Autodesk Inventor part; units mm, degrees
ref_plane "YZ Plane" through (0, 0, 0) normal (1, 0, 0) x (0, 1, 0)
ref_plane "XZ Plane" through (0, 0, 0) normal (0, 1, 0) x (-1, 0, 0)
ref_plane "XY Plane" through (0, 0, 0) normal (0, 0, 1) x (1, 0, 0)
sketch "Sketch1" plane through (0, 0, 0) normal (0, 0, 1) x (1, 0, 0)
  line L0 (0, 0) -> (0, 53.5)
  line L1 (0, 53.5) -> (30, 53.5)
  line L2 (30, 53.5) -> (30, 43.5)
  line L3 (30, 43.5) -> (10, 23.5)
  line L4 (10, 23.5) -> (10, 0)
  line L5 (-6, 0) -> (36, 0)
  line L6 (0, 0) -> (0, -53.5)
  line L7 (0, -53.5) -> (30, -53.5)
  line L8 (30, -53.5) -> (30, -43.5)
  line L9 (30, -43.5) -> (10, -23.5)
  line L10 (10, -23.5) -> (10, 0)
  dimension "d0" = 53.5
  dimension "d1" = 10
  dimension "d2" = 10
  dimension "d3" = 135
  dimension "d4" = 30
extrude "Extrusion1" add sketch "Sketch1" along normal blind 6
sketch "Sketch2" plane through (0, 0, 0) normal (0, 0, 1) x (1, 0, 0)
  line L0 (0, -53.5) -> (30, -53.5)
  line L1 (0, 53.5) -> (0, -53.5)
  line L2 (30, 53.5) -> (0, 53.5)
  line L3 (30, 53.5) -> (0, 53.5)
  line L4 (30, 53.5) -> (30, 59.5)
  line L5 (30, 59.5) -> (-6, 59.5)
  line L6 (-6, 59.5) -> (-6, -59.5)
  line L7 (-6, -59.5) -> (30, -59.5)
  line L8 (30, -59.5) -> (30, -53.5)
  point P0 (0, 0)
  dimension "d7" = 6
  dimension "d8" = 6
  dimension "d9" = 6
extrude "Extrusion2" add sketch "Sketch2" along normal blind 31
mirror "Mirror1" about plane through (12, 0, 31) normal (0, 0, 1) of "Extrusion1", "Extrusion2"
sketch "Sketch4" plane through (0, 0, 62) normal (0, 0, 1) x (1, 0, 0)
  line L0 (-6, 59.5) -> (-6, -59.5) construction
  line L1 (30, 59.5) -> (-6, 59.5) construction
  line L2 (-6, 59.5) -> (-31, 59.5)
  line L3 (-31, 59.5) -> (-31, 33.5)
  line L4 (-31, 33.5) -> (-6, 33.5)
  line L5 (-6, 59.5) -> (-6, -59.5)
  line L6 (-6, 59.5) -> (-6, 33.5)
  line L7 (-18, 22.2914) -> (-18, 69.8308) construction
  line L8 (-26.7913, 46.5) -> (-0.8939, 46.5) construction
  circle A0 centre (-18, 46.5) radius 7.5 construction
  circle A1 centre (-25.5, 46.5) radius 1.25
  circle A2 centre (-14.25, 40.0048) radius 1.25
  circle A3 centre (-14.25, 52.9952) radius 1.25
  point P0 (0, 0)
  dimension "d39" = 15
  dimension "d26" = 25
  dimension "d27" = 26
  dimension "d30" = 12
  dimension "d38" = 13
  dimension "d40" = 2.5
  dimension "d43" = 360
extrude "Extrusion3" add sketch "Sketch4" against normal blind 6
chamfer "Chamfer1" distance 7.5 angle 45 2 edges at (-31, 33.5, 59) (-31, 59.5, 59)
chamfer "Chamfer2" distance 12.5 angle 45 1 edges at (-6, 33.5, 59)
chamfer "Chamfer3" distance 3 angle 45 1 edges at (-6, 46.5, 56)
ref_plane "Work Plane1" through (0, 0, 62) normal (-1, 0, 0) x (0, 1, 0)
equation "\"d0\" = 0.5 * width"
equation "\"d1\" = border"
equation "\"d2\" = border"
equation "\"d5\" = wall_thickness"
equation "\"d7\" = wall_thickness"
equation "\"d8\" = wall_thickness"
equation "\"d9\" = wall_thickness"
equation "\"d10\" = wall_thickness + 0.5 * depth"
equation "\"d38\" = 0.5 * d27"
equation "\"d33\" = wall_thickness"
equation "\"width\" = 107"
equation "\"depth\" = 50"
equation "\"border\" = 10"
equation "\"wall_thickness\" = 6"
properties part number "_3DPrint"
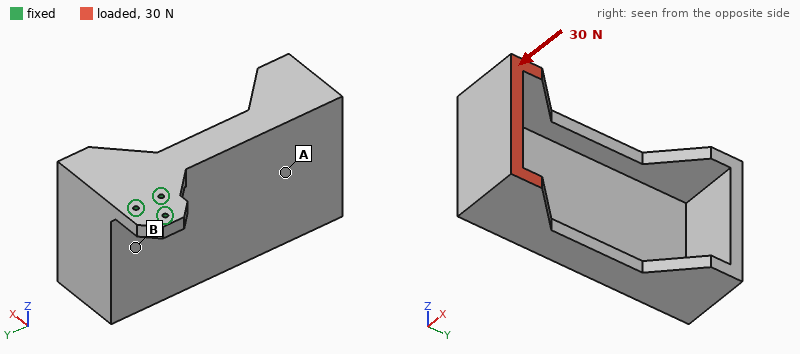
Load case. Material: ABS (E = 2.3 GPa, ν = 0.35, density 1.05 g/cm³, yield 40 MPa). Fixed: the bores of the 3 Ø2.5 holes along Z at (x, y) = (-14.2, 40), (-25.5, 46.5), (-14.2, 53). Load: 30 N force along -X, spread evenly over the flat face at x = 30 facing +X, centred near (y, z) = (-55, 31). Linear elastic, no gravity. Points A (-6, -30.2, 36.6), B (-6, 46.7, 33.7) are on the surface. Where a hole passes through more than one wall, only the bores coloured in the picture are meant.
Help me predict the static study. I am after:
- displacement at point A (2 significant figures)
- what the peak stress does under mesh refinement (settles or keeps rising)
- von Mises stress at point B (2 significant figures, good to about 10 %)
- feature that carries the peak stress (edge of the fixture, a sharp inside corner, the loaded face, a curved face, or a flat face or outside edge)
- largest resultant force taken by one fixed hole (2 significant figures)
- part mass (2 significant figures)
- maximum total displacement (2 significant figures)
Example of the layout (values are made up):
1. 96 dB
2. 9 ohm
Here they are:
1. 0.78 mm
2. keeps rising
3. 1.5 MPa
4. edge of the fixture
5. 170 N
6. 98 g
7. 1.8 mm
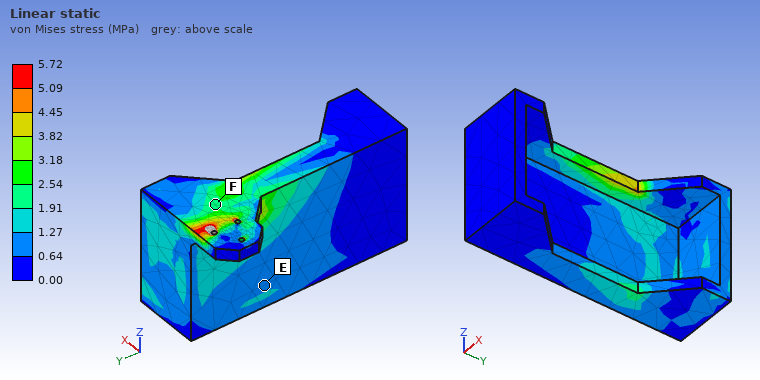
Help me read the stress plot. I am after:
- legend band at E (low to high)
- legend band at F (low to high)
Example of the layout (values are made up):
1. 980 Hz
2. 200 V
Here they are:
1. 0.64 to 1.27 MPa
2. 1.91 to 2.54 MPa
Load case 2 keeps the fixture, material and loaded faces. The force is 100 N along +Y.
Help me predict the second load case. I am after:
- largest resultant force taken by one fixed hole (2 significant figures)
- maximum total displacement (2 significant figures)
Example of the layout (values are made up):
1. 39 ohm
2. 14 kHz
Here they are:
1. 300 N
2. 1.8 mm
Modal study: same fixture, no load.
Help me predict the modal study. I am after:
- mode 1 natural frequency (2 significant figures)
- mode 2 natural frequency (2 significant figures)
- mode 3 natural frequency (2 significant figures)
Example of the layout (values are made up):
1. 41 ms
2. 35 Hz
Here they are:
1. 110 Hz
2. 150 Hz
3. 240 Hz
